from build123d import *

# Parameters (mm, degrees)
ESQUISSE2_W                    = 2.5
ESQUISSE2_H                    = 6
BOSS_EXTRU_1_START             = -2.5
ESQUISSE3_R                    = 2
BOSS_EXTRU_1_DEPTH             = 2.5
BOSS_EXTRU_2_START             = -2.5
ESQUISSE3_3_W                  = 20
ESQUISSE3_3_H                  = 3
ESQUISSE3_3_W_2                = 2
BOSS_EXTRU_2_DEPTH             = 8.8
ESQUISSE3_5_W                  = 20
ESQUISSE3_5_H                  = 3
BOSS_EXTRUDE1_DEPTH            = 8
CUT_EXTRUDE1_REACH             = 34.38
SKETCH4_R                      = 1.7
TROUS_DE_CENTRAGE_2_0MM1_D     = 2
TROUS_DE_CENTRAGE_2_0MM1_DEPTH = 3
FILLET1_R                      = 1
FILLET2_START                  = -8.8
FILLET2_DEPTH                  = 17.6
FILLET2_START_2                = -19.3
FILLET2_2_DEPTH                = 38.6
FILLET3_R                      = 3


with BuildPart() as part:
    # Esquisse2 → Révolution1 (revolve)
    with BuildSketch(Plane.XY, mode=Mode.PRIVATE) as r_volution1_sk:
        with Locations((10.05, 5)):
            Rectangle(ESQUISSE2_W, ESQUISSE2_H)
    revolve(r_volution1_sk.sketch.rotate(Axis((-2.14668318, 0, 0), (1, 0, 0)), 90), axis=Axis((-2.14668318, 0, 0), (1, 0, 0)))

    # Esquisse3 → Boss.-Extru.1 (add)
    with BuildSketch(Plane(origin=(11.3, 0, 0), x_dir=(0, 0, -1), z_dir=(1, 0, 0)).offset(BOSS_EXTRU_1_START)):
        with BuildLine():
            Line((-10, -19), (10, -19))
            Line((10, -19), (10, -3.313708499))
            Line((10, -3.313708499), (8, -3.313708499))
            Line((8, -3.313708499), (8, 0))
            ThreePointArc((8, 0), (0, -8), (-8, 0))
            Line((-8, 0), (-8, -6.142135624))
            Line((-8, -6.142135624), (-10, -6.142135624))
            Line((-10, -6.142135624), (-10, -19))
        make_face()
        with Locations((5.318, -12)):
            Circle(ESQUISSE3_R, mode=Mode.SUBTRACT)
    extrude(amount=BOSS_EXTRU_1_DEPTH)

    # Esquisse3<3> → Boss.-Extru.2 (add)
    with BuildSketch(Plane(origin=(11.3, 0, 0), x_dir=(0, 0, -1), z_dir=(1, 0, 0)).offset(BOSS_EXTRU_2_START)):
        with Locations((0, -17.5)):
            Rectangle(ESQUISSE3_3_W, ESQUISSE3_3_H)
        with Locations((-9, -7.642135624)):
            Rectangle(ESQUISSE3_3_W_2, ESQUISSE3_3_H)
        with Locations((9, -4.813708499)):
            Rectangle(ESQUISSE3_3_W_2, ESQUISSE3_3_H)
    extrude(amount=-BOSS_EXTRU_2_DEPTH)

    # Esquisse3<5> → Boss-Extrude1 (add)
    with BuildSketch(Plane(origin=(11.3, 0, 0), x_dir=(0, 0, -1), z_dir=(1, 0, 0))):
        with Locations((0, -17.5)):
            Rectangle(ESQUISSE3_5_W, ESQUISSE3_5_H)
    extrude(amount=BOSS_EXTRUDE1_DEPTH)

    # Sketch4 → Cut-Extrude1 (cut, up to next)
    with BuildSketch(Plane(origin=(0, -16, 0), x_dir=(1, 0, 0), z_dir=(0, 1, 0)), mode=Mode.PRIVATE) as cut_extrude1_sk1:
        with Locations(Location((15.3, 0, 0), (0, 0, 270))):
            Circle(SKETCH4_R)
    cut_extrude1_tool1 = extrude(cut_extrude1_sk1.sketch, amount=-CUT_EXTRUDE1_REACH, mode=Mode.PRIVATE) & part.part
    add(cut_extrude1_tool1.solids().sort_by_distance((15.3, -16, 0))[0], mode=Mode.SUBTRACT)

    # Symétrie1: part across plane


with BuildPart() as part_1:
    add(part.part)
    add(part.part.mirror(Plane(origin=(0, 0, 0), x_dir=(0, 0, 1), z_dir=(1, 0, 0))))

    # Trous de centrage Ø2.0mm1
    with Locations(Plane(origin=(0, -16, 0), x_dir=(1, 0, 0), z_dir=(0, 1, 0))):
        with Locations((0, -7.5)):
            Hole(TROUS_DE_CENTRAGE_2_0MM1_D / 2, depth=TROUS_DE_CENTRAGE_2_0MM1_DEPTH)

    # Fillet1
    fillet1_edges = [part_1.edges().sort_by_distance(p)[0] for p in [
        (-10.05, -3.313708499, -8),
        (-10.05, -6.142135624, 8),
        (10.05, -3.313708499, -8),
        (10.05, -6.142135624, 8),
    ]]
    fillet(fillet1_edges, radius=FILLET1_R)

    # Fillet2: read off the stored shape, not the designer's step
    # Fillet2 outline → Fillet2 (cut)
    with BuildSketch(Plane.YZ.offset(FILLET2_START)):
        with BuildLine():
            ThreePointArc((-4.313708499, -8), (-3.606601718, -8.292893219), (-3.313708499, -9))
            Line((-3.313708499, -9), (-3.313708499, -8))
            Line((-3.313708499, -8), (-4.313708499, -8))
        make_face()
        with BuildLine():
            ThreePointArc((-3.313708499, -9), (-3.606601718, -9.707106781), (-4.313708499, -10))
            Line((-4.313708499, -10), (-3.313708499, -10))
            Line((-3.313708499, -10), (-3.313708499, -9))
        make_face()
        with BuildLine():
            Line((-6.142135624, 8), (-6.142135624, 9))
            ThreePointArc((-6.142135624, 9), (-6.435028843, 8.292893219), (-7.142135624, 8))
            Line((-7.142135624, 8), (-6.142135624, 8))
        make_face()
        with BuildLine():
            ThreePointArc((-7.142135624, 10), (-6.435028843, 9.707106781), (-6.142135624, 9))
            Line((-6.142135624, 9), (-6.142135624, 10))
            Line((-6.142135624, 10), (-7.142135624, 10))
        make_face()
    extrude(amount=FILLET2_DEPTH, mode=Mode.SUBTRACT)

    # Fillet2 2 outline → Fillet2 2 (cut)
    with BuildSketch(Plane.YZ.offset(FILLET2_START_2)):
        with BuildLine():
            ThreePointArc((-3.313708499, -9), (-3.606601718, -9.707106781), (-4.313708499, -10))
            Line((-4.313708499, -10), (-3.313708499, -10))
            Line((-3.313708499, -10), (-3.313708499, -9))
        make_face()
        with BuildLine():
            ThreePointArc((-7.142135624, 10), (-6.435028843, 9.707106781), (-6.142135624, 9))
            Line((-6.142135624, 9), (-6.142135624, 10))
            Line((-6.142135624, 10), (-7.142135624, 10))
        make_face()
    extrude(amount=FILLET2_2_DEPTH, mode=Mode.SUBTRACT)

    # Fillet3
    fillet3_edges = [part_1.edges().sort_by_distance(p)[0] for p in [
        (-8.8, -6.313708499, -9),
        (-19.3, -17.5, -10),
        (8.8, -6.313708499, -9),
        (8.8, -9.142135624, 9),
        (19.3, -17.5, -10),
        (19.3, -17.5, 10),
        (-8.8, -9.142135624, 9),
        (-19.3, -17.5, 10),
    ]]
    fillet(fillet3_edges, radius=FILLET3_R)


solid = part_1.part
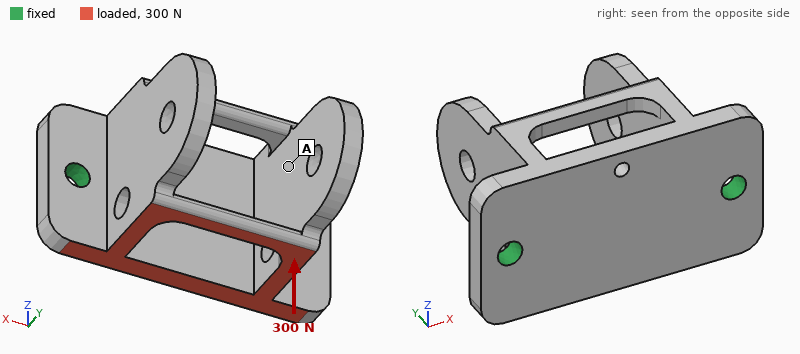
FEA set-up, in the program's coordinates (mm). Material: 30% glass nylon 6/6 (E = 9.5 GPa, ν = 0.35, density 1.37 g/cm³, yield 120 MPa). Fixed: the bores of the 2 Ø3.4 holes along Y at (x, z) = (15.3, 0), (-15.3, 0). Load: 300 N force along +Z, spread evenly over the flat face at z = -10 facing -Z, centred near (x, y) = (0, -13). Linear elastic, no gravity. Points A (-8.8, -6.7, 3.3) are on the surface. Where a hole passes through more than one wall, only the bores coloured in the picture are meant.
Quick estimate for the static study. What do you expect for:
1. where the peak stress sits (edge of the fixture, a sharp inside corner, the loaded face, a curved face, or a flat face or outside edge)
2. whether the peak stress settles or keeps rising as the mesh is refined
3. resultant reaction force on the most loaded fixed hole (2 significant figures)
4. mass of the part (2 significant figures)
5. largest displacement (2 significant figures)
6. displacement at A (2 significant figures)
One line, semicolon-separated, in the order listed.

edge of the fixture; keeps rising; 150 N; 5.9 g; 0.18 mm; 0.067 mm
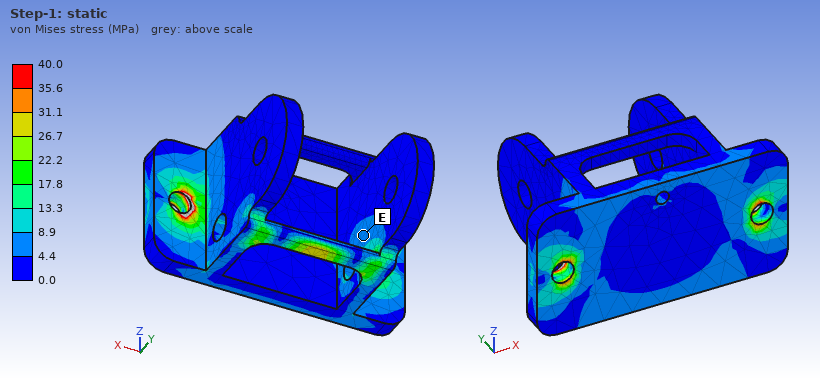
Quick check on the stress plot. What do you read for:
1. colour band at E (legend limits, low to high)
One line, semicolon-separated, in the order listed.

4.4 to 8.9 MPa
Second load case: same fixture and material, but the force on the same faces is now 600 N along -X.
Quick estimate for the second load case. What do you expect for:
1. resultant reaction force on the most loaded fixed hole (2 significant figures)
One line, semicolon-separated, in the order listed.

360 N
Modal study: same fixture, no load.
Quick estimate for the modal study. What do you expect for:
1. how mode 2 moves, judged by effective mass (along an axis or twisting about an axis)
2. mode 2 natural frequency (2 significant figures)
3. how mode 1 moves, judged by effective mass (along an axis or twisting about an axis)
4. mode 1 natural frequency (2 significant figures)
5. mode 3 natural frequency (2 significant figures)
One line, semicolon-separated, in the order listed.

along Z; 3000 Hz; along X; 2700 Hz; 3700 Hz
